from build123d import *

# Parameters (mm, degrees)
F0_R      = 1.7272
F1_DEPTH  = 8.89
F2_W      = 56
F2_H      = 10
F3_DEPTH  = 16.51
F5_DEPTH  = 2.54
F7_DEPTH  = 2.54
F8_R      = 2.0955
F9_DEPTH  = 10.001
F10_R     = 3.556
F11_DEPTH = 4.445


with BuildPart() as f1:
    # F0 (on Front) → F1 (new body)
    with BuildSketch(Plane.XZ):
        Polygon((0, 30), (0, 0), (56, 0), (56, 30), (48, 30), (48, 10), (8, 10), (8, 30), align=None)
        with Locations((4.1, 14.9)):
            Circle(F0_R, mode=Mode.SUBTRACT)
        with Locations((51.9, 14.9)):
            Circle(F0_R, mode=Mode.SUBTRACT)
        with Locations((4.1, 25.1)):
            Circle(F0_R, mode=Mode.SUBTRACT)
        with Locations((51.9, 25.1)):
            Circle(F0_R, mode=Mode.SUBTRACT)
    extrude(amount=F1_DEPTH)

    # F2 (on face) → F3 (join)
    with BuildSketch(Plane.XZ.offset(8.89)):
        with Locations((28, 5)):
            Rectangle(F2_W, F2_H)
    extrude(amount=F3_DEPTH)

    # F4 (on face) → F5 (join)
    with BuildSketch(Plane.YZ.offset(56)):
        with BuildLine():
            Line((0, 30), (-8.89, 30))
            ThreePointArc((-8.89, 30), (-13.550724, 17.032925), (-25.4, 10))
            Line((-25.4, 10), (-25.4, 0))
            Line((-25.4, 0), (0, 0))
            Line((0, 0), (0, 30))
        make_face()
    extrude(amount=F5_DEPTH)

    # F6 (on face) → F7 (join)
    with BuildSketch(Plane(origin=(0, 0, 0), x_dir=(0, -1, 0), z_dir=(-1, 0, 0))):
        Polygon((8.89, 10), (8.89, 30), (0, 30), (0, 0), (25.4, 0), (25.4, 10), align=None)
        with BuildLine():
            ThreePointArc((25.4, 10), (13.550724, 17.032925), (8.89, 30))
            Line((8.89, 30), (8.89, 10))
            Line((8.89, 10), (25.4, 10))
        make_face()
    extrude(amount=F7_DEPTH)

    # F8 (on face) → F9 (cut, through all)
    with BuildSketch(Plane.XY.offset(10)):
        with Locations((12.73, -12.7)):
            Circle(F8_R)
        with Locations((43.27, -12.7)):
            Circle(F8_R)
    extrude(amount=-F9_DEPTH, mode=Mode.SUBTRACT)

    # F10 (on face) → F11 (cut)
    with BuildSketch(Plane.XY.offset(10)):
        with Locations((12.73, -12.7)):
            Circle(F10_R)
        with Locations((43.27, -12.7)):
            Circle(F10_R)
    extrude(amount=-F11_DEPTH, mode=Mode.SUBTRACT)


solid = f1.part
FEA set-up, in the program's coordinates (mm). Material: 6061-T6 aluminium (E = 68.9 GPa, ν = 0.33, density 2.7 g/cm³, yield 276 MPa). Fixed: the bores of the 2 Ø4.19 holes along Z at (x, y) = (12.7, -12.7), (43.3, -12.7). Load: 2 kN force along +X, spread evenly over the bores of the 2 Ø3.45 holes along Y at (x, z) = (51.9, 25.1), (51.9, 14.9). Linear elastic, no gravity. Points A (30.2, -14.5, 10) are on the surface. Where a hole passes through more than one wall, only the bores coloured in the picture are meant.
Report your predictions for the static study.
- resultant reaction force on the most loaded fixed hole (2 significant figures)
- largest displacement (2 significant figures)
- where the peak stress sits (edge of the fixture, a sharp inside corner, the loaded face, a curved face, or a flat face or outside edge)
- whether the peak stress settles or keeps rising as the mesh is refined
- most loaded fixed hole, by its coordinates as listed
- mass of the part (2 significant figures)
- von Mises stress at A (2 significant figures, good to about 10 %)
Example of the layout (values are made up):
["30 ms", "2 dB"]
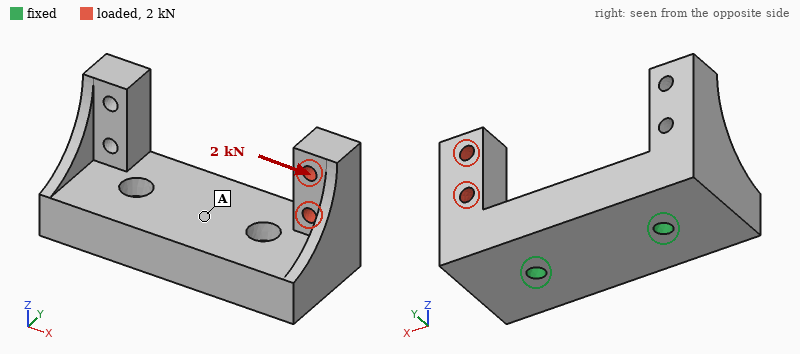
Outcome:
["1.8 kN", "0.19 mm", "edge of the fixture", "keeps rising", "(12.7, -12.7)", "51 g", "23 MPa"]
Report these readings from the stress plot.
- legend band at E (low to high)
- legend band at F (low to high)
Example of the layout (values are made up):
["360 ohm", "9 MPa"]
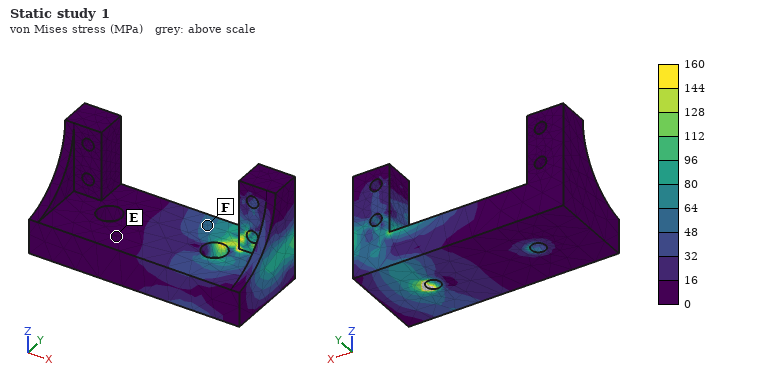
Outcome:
["0 to 16 MPa", "48 to 64 MPa"]
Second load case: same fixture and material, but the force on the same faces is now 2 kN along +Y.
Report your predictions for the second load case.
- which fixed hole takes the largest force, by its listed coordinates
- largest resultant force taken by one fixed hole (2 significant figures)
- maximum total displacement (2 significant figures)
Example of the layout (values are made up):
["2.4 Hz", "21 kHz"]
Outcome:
["(43.3, -12.7)", "2.4 kN", "0.22 mm"]
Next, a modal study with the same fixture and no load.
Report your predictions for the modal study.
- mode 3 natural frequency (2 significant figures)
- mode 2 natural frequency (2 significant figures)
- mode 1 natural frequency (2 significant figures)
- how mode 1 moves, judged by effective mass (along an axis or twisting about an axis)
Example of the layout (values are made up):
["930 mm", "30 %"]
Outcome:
["8500 Hz", "7500 Hz", "6700 Hz", "along Y"]
